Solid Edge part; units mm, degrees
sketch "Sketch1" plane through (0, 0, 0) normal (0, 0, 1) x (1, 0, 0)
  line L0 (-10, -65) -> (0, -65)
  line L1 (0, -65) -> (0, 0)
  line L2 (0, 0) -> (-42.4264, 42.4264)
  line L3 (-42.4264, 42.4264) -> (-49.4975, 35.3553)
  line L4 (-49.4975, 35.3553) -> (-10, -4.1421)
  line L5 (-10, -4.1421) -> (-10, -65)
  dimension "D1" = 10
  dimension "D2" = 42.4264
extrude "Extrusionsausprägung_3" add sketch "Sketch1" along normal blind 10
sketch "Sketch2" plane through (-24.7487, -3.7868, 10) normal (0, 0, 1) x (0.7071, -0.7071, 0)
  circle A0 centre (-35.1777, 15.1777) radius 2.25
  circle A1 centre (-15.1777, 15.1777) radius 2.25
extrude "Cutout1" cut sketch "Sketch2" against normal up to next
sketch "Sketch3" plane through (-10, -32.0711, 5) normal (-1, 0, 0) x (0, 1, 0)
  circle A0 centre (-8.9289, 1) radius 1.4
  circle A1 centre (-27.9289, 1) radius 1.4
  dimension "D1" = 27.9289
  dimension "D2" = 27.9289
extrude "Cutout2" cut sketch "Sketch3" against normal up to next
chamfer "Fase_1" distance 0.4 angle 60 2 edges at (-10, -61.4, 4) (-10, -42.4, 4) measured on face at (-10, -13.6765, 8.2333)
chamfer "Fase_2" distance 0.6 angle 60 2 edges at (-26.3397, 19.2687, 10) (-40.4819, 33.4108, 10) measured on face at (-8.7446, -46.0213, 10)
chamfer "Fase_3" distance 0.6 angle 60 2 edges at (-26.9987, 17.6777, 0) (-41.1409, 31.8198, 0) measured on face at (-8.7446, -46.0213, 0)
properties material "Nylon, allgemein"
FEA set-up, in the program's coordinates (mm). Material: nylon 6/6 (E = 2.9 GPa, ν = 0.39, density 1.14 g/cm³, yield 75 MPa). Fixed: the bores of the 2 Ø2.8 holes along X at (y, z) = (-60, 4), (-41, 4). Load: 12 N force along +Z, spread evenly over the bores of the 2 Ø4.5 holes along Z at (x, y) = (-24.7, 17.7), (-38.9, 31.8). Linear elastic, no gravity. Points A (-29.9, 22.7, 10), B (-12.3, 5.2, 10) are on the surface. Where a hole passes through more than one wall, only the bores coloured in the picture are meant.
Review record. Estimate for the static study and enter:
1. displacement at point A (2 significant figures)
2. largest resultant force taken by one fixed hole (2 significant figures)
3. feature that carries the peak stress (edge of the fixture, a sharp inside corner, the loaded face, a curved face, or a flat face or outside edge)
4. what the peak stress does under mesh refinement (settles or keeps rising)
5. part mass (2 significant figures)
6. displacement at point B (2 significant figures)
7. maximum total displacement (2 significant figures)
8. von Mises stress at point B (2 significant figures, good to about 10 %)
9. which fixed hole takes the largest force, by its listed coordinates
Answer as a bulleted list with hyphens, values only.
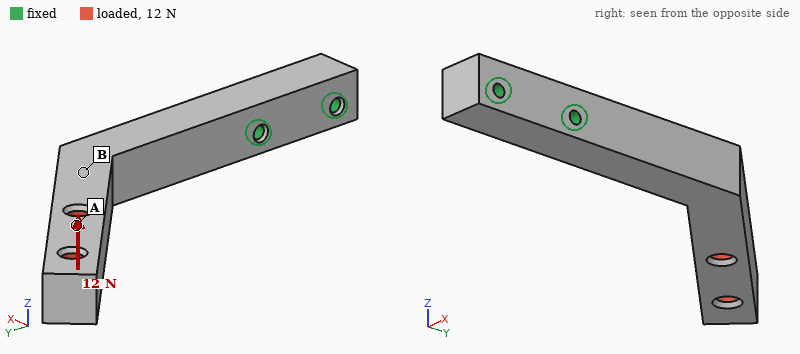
- 0.79 mm
- 43 N
- edge of the fixture
- keeps rising
- 13 g
- 0.40 mm
- 1.2 mm
- 2.0 MPa
- (-41, 4)
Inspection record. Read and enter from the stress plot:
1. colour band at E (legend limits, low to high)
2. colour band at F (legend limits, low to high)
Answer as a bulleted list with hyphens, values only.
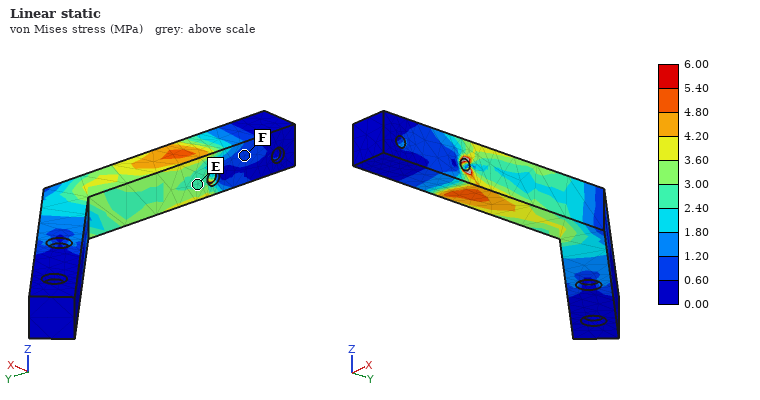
- 2.40 to 3.00 MPa
- 0.60 to 1.20 MPa
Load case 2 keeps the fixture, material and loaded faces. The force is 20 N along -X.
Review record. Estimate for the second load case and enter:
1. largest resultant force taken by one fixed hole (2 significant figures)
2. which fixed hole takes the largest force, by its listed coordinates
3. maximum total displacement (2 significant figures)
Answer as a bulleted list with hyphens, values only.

- 33 N
- (-41, 4)
- 1.4 mm
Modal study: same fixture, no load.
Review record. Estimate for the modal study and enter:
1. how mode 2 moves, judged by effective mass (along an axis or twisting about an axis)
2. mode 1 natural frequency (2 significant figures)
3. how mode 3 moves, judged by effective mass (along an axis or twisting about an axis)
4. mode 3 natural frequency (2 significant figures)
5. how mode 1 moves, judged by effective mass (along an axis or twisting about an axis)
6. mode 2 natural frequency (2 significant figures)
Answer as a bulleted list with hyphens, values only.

- along X
- 270 Hz
- along Z
- 1200 Hz
- along Z
- 300 Hz
